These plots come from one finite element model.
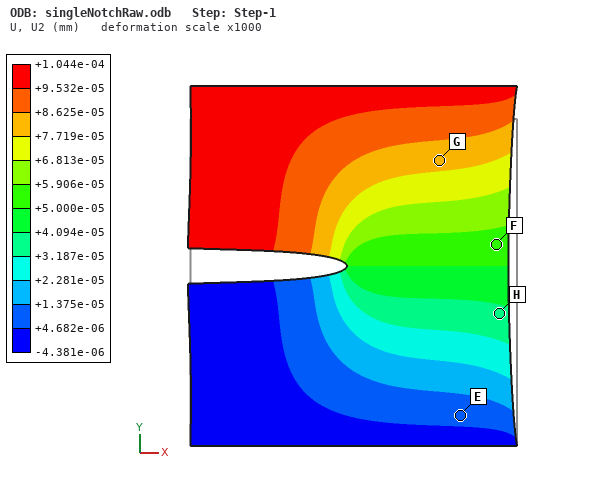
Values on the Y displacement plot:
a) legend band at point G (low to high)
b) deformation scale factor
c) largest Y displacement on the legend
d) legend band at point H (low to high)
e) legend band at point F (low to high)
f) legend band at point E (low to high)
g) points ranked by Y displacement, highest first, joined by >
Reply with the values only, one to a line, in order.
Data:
+7.719e-05 to +8.625e-05 mm
1000
+1.044e-04 mm
+3.187e-05 to +4.094e-05 mm
+5.000e-05 to +5.906e-05 mm
+4.682e-06 to +1.375e-05 mm
G > F > H > E
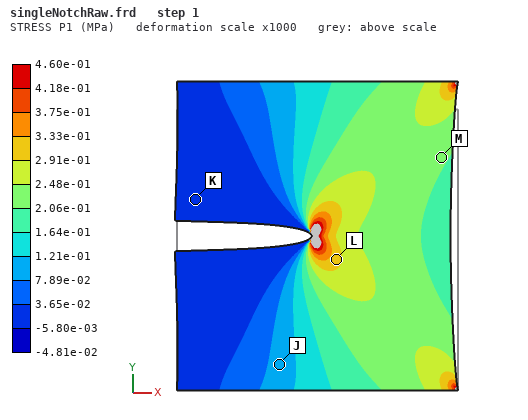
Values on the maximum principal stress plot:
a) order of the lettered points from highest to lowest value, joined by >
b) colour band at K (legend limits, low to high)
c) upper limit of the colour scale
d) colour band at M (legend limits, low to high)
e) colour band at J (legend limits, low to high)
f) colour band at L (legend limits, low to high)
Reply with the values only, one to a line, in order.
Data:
L > M > J > K
-5.80e-03 to 3.65e-02 MPa
4.60e-01 MPa
2.06e-01 to 2.48e-01 MPa
7.89e-02 to 1.21e-01 MPa
2.91e-01 to 3.33e-01 MPa
